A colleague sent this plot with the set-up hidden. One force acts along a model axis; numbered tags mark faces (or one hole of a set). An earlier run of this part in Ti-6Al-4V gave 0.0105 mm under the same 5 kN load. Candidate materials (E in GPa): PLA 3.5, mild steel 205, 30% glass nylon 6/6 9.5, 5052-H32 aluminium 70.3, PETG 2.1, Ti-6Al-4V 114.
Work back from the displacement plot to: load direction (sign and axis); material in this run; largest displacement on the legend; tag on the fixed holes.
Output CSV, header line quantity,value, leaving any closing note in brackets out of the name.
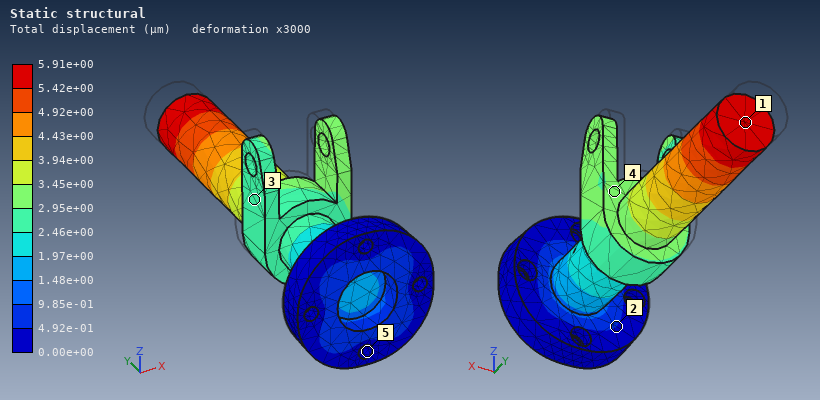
quantity,value
load direction,-Y
material in this run,mild steel
largest displacement on the legend,5.91e+00 µm
tag on the fixed holes,5
